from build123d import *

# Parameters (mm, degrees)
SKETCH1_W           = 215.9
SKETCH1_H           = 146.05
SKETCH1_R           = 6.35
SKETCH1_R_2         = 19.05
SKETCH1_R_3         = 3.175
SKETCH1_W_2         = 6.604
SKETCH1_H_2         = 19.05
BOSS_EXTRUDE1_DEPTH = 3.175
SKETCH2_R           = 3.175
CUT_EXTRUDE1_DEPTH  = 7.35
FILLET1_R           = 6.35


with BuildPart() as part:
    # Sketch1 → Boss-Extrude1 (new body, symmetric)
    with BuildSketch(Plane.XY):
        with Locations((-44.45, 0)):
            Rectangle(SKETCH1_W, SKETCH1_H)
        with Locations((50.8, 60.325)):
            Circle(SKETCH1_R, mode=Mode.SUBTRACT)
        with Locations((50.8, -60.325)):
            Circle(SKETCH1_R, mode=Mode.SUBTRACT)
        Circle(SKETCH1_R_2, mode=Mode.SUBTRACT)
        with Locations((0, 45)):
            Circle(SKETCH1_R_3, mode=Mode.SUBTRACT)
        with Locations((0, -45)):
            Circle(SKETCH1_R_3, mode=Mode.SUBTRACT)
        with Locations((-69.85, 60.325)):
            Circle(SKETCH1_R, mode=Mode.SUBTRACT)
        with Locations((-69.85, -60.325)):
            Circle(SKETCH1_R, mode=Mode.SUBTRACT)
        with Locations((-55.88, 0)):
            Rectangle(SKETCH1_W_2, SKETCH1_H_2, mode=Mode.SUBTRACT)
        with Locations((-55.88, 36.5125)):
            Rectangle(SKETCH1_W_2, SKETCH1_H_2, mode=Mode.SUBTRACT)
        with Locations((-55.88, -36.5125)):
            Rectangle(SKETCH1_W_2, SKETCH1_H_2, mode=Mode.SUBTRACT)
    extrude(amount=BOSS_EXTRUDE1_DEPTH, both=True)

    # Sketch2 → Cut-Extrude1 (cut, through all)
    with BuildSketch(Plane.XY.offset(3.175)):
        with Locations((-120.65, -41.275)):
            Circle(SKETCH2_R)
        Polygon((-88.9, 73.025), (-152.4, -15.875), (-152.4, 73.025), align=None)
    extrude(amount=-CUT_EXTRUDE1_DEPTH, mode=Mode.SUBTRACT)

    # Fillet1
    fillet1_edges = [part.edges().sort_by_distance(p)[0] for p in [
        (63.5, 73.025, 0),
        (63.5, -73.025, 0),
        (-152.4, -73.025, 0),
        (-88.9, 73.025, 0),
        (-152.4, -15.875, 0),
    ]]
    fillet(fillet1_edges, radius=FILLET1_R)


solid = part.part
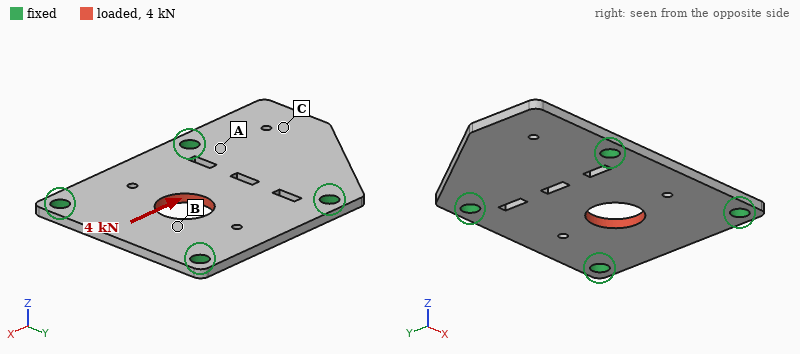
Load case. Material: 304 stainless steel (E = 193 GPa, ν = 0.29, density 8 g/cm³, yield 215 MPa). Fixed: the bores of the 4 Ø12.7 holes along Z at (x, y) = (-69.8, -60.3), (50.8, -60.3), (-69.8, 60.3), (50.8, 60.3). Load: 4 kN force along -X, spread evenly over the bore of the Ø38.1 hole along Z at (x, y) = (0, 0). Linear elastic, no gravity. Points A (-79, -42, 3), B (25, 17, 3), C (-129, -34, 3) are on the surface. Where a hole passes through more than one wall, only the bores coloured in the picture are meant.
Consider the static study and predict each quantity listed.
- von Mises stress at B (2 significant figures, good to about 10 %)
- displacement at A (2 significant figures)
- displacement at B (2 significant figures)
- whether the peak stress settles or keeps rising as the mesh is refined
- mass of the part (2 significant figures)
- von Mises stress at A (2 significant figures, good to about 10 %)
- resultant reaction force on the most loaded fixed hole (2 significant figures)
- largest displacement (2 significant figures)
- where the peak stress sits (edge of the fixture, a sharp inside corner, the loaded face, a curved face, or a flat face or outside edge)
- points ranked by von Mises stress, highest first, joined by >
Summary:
4.6 MPa
0.41 µm
2.0 µm
keeps rising
1.3 kg
2.3 MPa
1.1 kN
2.6 µm
edge of the fixture
B > A > C
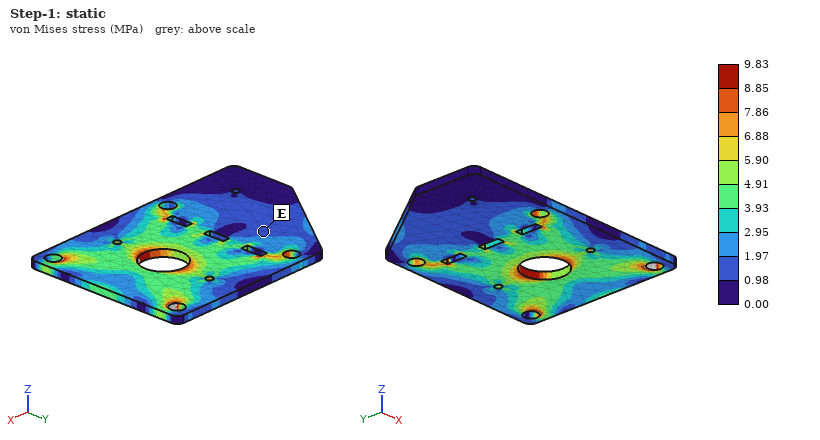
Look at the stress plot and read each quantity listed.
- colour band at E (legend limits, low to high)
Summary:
0.98 to 1.97 MPa
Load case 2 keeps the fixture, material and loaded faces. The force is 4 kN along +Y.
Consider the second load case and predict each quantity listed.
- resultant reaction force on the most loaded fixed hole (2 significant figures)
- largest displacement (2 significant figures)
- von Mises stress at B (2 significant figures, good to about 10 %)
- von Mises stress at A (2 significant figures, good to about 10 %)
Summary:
1.3 kN
2.5 µm
5.3 MPa
1.9 MPa
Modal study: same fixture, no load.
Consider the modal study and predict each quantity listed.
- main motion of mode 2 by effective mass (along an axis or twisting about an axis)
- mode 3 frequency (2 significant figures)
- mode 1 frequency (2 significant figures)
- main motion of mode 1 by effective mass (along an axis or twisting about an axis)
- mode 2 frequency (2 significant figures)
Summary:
along Z
1800 Hz
790 Hz
along Z
1700 Hz
